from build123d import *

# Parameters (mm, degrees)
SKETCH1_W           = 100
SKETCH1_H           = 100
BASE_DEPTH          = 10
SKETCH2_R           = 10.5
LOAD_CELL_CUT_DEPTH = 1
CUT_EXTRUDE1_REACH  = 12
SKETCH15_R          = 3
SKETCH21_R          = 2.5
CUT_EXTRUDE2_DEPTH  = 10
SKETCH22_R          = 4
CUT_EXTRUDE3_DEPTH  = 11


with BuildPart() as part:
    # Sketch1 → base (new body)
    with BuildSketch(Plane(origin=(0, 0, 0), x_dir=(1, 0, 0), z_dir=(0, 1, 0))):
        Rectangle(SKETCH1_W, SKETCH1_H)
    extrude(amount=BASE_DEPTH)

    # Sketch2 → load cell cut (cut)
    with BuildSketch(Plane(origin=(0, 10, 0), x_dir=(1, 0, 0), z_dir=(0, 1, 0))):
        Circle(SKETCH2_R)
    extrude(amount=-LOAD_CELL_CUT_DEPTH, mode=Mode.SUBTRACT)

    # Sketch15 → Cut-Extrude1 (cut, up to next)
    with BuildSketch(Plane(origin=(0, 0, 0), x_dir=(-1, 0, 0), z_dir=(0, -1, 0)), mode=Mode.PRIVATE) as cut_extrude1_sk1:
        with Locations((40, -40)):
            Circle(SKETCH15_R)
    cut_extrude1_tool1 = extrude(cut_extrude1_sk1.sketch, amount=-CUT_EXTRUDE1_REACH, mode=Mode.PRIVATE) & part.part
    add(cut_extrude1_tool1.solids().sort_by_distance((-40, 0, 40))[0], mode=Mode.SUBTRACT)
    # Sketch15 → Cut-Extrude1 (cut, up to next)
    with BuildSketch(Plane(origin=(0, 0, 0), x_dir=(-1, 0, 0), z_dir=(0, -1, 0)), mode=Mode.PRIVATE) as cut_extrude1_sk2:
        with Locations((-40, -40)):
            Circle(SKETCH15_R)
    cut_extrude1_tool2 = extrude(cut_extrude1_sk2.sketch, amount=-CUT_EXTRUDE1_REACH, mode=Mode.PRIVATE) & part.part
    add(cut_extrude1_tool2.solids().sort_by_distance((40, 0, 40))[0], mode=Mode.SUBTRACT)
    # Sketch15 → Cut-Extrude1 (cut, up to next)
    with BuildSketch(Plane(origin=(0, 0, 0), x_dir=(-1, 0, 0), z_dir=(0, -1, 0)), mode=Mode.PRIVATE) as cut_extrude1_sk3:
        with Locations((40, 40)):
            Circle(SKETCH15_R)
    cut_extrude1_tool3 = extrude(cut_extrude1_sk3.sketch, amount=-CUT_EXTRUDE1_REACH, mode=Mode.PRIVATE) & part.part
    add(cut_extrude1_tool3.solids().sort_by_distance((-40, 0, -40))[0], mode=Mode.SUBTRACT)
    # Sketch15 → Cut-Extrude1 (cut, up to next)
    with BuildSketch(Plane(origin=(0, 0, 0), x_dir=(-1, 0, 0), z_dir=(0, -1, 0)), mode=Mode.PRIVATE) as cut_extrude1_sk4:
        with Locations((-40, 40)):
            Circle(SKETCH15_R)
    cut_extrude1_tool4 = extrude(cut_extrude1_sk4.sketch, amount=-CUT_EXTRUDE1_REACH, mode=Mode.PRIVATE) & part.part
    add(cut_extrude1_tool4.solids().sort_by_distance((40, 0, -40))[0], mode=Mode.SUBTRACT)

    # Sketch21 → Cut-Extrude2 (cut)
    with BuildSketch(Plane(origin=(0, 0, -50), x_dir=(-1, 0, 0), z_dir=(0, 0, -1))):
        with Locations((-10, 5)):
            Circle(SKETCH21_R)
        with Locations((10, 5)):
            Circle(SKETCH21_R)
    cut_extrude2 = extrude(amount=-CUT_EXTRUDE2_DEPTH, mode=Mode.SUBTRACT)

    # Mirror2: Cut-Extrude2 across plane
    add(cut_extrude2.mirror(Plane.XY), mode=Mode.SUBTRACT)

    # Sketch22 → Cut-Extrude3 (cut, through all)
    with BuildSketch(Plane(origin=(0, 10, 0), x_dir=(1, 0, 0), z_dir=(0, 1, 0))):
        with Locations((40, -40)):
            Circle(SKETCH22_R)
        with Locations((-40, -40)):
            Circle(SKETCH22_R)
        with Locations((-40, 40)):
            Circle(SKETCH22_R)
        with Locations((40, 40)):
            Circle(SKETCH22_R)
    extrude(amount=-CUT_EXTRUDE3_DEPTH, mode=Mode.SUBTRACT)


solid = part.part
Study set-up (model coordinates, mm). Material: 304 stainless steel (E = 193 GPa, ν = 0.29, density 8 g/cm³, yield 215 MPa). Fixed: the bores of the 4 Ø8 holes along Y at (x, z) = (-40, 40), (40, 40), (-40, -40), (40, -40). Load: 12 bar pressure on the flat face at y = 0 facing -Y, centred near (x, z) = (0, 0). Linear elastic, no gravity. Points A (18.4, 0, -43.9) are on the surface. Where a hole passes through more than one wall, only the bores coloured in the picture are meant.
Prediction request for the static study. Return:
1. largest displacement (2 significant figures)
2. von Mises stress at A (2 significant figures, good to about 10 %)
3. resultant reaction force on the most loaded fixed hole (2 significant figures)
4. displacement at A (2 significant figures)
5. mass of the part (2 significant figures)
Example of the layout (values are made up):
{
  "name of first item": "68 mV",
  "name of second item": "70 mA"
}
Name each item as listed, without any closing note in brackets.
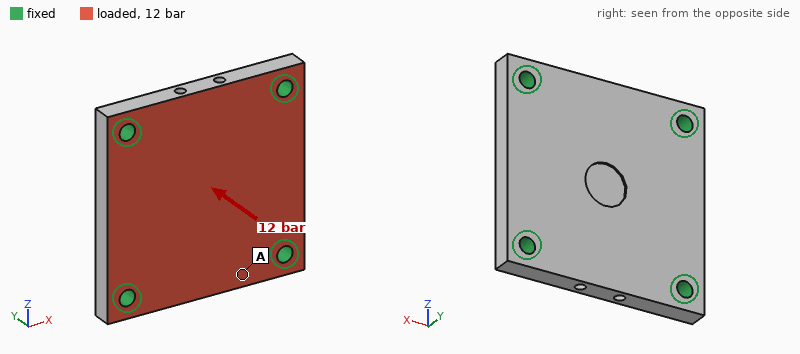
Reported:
{
  "largest displacement": "22 µm",
  "von Mises stress at A": "8.9 MPa",
  "resultant reaction force on the most loaded fixed hole": "2.9 kN",
  "displacement at A": "7.0 µm",
  "mass of the part": "770 g"
}
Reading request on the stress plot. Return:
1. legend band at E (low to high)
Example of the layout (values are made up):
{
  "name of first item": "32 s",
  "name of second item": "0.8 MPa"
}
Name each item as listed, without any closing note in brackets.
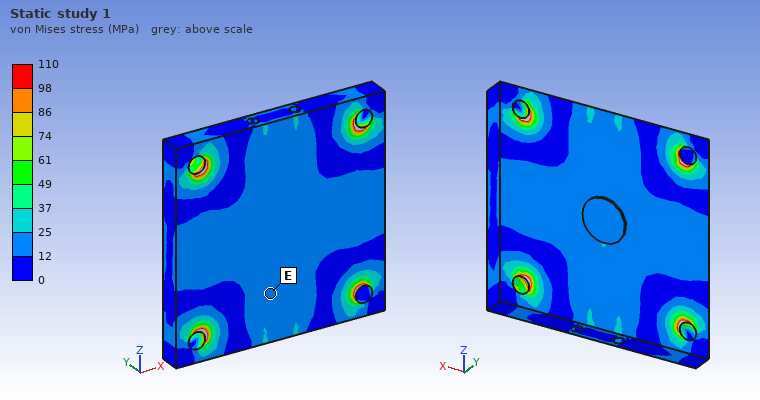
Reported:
{
  "legend band at E": "12 to 25 MPa"
}
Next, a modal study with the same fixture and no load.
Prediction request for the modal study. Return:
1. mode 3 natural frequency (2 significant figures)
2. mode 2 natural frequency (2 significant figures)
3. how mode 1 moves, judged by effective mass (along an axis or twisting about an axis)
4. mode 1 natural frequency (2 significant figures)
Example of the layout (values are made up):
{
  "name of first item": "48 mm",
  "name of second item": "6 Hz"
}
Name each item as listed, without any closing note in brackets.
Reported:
{
  "mode 3 natural frequency": "8300 Hz",
  "mode 2 natural frequency": "8200 Hz",
  "how mode 1 moves, judged by effective mass": "along Y",
  "mode 1 natural frequency": "5100 Hz"
}
